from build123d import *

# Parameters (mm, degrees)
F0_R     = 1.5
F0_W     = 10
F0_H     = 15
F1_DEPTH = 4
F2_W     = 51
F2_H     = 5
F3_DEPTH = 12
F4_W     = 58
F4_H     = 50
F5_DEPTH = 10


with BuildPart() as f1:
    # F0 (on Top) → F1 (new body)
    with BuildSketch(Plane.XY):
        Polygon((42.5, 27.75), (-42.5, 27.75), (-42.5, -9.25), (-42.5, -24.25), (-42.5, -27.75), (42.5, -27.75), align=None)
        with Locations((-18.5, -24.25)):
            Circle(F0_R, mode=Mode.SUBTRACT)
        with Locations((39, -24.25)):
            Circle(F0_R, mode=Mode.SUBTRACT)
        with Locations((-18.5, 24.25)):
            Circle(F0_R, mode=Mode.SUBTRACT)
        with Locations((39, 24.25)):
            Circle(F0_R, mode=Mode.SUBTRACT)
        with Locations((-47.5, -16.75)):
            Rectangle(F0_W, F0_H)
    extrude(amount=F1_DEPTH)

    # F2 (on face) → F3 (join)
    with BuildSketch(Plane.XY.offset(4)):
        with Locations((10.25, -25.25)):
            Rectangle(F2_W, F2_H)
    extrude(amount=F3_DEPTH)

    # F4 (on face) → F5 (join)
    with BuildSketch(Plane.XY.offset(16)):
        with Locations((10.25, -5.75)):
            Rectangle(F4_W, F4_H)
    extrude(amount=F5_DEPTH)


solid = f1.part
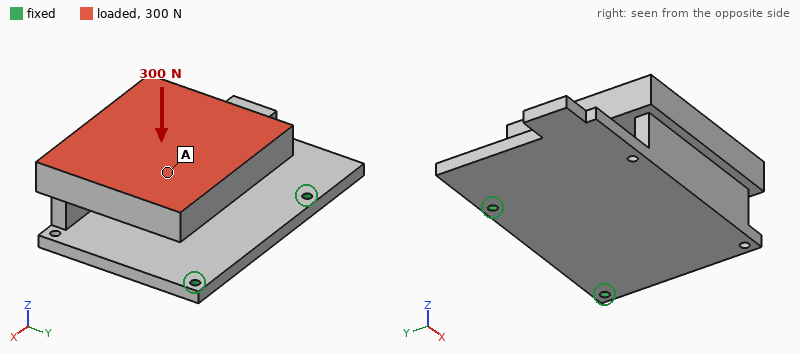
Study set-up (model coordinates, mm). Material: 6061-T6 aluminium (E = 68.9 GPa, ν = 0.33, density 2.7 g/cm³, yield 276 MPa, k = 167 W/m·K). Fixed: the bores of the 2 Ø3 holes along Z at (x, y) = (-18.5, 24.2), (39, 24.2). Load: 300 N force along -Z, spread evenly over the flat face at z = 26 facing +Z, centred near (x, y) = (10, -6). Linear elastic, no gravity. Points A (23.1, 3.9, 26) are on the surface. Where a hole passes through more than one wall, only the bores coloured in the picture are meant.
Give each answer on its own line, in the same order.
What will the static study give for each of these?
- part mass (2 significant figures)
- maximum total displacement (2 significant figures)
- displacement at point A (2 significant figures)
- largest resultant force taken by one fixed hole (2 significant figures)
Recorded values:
140 g
0.40 mm
0.27 mm
150 N
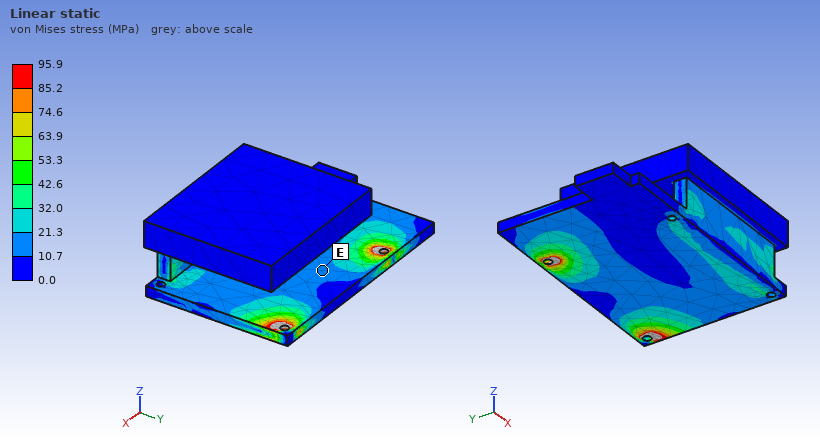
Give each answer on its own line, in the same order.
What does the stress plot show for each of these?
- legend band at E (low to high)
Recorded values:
10.7 to 21.3 MPa
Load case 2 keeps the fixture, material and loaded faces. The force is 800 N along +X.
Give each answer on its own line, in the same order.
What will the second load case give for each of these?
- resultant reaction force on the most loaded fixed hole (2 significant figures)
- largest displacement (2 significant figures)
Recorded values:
660 N
0.64 mm
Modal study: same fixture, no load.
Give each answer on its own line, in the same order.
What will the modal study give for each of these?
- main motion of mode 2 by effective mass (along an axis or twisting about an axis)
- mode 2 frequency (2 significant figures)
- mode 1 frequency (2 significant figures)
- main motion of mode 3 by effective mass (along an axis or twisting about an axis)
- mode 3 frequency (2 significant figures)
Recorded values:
along Z
660 Hz
390 Hz
along X
710 Hz
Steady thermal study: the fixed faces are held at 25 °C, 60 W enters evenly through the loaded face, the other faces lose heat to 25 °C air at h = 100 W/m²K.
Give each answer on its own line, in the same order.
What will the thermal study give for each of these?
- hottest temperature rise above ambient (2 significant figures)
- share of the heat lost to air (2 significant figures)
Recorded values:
50 K
70 %
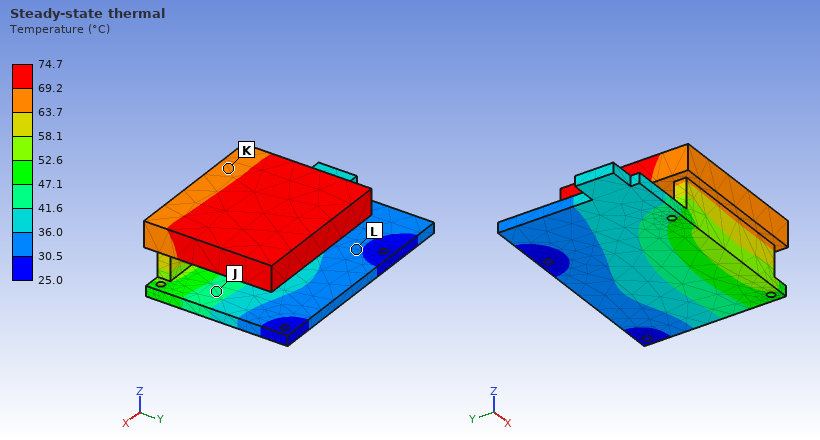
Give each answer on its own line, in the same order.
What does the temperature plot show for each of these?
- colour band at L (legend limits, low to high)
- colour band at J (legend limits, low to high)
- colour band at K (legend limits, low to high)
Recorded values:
30.5 to 36.0 °C
41.6 to 47.1 °C
63.7 to 69.2 °C
